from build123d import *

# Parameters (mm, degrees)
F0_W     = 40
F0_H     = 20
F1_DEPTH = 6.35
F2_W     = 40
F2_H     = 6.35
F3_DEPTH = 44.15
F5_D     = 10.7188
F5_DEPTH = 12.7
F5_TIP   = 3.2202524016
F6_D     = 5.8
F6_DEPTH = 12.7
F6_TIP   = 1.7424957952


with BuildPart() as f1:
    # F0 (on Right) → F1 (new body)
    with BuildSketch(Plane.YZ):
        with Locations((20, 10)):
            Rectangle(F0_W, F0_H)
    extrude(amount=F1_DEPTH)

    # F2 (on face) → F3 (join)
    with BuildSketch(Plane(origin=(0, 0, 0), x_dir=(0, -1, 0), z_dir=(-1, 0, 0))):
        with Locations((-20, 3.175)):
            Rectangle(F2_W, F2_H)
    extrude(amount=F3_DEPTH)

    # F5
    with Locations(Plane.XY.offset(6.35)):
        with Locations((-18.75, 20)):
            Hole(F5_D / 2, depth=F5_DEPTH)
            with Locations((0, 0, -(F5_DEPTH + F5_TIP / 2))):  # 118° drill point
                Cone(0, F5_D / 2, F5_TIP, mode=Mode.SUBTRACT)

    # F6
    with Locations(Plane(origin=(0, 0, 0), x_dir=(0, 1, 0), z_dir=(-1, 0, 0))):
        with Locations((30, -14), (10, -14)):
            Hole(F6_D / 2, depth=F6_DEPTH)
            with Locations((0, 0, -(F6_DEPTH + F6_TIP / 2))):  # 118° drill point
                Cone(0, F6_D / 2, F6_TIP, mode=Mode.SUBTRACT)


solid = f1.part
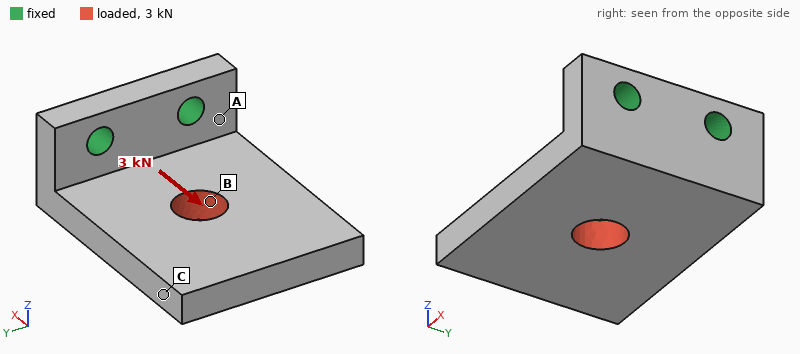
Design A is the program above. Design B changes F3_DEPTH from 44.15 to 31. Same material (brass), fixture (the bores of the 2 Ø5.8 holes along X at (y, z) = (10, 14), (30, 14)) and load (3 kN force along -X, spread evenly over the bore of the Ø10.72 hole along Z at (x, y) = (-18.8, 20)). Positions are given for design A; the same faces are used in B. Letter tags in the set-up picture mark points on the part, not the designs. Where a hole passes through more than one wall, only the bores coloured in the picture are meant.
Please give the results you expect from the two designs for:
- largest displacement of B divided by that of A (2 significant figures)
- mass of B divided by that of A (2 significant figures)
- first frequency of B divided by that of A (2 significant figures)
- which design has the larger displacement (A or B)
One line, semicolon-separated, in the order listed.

0.76; 0.78; 1.8; A
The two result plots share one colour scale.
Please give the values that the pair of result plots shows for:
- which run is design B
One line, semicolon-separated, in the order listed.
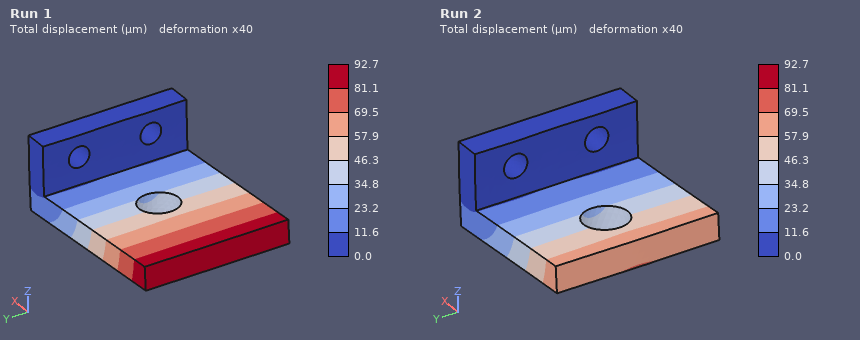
Run 2
